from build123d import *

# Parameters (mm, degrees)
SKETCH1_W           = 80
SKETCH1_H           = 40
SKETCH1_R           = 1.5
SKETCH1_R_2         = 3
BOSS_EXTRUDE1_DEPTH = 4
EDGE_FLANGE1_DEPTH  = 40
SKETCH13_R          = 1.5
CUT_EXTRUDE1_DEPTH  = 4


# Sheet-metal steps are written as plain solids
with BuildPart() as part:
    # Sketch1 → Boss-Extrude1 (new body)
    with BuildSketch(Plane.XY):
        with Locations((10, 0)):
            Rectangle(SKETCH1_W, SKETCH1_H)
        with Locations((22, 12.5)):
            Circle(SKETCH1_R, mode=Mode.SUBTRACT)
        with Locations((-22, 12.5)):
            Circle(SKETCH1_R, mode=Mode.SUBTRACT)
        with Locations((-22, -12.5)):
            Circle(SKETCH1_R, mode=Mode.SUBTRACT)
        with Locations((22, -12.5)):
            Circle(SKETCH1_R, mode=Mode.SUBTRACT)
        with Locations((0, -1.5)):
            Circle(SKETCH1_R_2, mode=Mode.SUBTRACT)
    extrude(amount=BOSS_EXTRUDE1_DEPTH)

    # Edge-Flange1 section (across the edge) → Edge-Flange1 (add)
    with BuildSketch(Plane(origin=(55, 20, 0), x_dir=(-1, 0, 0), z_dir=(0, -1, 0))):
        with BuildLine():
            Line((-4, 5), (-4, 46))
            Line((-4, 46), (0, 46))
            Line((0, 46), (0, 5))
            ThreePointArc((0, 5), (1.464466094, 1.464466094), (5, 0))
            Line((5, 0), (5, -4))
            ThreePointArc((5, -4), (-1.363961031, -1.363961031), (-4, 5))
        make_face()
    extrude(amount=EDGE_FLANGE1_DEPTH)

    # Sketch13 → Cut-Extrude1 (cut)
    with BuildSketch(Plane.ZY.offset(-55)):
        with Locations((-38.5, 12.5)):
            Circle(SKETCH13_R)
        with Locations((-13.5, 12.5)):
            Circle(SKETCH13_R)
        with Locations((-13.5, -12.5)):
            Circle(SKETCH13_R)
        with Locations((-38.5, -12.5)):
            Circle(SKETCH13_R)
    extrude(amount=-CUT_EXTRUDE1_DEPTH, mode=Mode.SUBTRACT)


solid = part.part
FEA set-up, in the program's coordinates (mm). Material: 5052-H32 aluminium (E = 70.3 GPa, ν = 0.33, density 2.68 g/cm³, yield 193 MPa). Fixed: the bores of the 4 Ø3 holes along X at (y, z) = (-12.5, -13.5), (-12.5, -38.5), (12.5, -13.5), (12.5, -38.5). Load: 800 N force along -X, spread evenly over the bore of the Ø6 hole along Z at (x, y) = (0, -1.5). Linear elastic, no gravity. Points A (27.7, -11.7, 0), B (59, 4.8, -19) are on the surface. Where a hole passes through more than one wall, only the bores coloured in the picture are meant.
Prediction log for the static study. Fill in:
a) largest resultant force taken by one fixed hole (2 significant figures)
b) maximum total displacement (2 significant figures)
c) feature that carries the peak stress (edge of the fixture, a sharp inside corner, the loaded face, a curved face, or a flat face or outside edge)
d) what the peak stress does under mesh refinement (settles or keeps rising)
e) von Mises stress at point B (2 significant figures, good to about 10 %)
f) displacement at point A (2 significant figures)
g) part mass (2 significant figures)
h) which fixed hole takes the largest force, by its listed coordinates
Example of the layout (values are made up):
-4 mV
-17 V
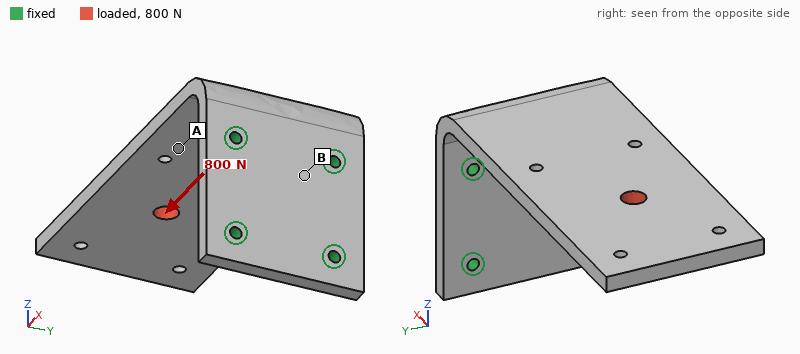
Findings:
520 N
0.62 mm
edge of the fixture
keeps rising
21 MPa
0.22 mm
56 g
(-12.5, -13.5)
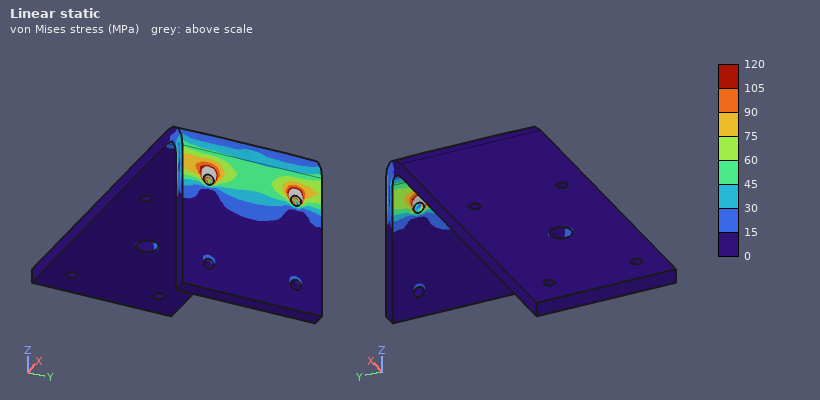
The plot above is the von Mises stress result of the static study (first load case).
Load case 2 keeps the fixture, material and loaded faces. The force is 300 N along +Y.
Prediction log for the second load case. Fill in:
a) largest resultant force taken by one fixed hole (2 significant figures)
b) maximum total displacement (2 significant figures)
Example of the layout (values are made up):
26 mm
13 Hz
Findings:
680 N
0.39 mm
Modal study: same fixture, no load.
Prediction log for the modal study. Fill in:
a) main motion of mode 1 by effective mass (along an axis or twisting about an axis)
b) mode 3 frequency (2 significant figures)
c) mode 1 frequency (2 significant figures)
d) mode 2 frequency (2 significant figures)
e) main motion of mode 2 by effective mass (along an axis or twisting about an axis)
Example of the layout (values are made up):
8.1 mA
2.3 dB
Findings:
along Z
2000 Hz
360 Hz
1000 Hz
along Y
